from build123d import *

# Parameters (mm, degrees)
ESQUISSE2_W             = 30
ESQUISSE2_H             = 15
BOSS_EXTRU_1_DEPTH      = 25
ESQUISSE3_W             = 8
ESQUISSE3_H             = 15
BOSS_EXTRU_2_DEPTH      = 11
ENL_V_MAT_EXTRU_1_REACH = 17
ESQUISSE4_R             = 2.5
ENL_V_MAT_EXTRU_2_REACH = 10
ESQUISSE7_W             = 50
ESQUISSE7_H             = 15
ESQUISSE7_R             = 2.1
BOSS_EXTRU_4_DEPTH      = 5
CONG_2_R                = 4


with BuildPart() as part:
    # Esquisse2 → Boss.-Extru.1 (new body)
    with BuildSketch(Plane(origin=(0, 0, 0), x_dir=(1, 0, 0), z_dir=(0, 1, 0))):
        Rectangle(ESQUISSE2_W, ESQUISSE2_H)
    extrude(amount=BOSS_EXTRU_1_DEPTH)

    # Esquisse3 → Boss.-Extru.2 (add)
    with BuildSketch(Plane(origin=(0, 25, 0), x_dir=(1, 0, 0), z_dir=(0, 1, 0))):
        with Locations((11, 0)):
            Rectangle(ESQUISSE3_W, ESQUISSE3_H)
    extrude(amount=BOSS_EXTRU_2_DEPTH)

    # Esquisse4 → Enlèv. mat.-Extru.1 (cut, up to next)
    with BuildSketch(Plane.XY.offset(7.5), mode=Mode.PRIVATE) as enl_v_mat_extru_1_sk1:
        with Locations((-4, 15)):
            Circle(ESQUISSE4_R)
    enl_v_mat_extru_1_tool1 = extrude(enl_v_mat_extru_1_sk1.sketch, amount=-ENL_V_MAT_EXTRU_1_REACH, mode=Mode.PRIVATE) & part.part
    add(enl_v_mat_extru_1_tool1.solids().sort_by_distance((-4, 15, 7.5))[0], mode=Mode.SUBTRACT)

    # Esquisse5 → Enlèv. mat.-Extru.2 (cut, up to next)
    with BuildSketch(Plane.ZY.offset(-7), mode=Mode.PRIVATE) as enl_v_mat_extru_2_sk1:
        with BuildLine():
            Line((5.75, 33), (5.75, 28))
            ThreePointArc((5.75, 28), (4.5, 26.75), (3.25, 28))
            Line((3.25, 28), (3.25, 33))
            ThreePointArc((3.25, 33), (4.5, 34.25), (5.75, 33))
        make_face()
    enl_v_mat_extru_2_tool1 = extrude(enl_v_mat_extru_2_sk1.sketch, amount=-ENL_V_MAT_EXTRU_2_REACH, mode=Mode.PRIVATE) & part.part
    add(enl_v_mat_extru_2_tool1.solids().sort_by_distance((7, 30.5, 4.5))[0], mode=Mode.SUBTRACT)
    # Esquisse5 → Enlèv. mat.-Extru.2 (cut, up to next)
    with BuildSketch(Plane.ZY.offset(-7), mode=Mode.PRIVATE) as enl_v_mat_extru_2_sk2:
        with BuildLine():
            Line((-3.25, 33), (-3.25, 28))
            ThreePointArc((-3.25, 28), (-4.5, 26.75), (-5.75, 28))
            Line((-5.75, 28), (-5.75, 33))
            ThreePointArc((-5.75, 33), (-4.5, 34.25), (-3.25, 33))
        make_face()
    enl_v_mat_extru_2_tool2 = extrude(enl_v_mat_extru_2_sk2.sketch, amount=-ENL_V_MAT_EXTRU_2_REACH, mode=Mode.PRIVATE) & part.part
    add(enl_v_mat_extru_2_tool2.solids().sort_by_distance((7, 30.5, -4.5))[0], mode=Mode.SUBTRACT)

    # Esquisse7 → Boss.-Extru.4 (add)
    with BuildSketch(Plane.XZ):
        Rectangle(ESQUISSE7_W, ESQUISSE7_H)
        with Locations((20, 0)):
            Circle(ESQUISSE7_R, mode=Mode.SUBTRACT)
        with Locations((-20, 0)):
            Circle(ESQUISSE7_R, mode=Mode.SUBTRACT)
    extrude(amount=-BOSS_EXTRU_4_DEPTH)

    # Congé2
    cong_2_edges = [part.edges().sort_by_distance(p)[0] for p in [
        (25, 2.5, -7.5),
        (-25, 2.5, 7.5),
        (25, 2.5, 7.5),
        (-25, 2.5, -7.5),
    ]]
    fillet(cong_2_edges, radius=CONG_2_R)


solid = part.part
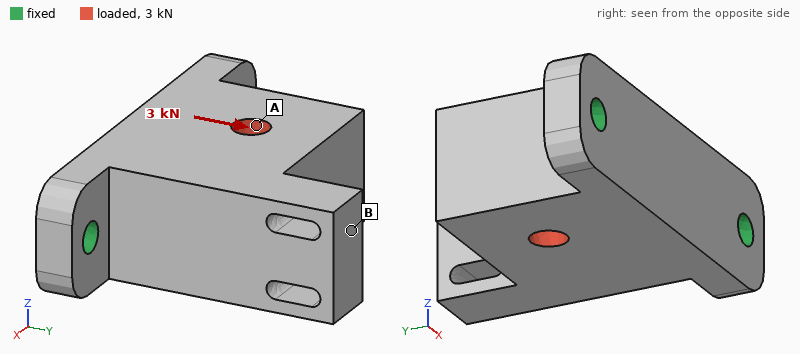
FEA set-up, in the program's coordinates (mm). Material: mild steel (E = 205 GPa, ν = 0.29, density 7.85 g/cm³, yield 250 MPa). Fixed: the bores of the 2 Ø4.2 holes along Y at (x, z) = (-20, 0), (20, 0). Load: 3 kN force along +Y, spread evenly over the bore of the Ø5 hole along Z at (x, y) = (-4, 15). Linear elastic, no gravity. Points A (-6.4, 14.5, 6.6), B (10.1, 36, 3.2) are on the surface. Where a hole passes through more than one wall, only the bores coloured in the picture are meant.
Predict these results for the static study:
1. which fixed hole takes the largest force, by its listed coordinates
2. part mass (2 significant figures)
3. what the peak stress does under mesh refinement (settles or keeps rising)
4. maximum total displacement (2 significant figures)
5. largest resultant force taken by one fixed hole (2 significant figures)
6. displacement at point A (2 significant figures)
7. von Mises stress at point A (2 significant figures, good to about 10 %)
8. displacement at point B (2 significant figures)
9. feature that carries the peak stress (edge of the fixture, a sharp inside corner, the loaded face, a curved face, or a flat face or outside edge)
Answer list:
(-20, 0)
100 g
keeps rising
5.1 µm
2.0 kN
4.9 µm
23 MPa
4.3 µm
edge of the fixture
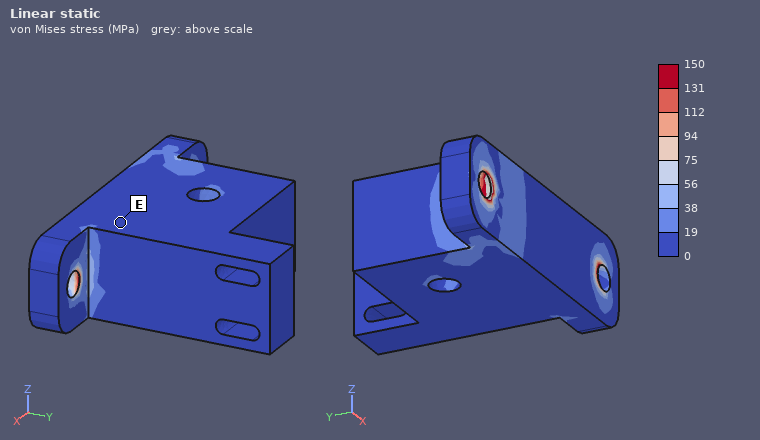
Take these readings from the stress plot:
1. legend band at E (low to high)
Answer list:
0 to 19 MPa
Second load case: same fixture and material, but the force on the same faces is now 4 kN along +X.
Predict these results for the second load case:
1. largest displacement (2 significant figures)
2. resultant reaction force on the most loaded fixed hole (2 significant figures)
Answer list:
9.9 µm
2.5 kN
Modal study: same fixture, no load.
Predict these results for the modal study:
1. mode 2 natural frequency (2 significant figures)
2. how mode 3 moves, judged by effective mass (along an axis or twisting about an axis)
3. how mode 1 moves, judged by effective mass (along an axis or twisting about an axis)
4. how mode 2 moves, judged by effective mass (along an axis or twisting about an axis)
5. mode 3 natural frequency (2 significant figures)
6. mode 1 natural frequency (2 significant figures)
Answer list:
12 kHz
along Y
along Z
along X
14 kHz
4100 Hz
